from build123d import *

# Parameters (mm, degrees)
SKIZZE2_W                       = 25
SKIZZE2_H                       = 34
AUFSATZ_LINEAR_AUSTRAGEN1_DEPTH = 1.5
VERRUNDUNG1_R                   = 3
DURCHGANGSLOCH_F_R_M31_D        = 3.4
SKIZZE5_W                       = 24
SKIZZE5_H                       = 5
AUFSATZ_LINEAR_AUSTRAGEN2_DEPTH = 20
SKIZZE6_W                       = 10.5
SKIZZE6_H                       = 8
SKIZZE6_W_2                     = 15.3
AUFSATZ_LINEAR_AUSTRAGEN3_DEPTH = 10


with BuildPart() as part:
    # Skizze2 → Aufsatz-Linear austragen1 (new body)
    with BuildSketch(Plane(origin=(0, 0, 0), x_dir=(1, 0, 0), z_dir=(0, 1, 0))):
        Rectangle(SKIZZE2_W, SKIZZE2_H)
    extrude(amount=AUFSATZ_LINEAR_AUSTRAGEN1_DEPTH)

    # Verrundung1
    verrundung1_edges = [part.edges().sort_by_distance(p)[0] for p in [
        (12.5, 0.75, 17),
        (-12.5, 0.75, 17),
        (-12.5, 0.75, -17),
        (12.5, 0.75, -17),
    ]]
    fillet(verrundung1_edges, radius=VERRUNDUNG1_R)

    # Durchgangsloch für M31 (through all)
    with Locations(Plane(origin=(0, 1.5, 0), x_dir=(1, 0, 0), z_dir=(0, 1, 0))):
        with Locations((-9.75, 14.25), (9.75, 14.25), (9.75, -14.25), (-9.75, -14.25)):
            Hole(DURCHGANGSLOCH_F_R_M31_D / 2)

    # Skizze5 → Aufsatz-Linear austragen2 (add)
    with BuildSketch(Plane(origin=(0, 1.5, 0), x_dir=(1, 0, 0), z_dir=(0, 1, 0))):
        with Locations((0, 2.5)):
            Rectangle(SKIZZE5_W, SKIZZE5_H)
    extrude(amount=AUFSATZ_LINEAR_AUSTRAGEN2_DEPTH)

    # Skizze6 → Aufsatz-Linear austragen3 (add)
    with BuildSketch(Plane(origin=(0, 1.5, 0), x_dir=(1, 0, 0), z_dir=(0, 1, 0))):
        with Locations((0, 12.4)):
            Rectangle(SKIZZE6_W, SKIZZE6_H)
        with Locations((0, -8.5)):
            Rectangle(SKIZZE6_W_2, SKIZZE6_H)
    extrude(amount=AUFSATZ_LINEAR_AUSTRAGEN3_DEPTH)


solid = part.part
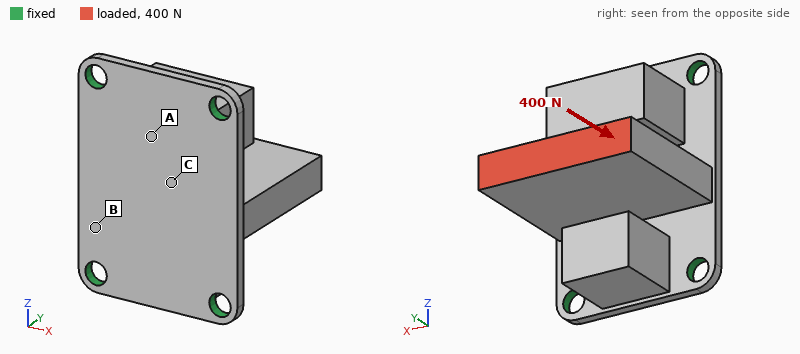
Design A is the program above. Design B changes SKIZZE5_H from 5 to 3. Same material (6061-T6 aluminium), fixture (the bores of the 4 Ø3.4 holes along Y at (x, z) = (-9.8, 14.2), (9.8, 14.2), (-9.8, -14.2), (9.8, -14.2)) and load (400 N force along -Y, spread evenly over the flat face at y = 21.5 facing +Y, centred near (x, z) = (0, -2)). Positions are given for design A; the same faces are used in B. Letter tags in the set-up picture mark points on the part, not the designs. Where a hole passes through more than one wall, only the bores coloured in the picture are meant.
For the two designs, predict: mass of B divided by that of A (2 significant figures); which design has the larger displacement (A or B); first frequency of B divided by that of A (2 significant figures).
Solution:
0.83
B
1.0
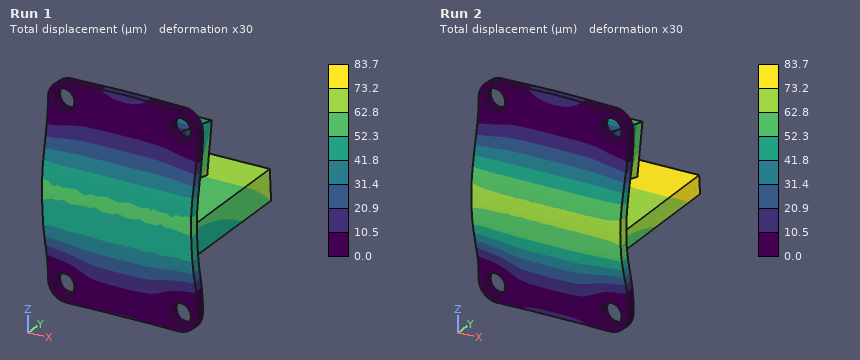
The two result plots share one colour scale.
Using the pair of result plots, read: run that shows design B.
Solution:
Run 2
